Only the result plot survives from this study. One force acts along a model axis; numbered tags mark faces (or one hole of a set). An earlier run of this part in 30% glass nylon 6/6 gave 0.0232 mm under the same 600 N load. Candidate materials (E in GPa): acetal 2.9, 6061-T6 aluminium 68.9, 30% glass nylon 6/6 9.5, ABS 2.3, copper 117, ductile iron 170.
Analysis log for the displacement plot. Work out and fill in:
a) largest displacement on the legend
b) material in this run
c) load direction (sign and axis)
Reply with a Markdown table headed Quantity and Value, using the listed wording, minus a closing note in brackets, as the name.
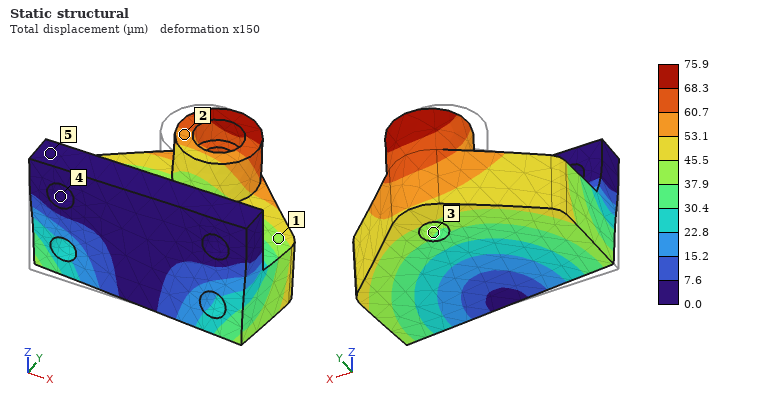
| Quantity | Value |
|---|---|
| largest displacement on the legend | 75.9 µm |
| material in this run | acetal |
| load direction | +X |
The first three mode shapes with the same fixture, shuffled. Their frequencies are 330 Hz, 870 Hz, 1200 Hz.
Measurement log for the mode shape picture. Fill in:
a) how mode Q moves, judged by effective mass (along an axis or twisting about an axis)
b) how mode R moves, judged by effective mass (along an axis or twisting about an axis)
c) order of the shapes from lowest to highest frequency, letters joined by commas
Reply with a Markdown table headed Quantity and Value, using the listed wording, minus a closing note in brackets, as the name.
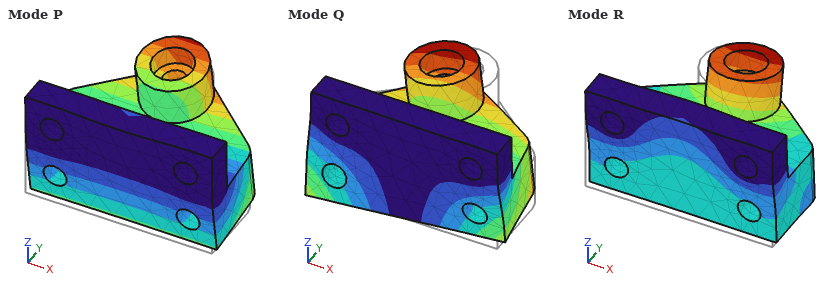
| Quantity | Value |
|---|---|
| how mode Q moves, judged by effective mass | along X |
| how mode R moves, judged by effective mass | along Y |
| order of the shapes from lowest to highest frequency, letters joined by commas | P, Q, R |
